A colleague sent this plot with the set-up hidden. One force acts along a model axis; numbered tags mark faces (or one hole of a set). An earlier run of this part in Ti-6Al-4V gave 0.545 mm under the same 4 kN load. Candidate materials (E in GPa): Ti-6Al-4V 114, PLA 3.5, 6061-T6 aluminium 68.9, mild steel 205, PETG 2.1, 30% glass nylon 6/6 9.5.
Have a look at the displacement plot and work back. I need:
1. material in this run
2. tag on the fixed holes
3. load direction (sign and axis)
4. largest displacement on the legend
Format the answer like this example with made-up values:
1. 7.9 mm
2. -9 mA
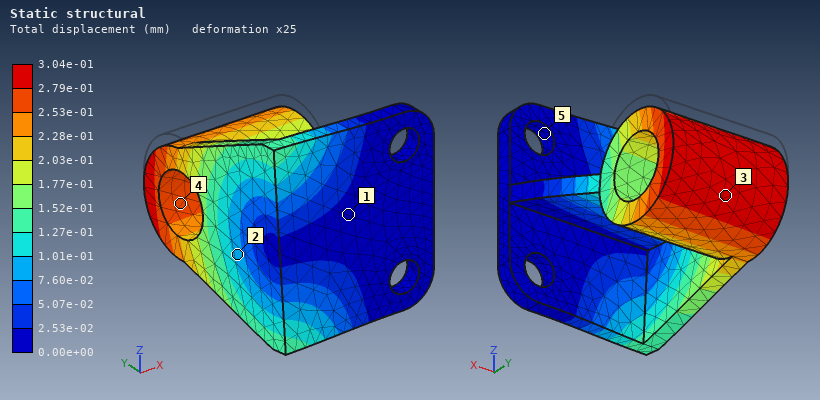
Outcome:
1. mild steel
2. 5
3. -Z
4. 3.04e-01 mm
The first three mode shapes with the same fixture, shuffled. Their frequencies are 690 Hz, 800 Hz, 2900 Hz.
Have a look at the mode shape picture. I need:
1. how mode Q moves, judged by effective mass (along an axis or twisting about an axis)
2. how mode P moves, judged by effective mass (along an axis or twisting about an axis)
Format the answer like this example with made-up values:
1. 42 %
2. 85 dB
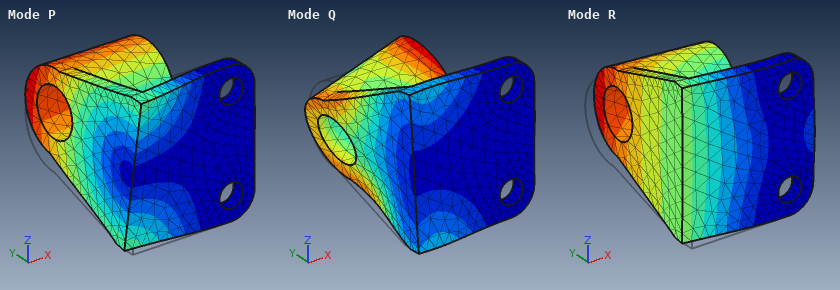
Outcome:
1. twisting about Y
2. along Z
